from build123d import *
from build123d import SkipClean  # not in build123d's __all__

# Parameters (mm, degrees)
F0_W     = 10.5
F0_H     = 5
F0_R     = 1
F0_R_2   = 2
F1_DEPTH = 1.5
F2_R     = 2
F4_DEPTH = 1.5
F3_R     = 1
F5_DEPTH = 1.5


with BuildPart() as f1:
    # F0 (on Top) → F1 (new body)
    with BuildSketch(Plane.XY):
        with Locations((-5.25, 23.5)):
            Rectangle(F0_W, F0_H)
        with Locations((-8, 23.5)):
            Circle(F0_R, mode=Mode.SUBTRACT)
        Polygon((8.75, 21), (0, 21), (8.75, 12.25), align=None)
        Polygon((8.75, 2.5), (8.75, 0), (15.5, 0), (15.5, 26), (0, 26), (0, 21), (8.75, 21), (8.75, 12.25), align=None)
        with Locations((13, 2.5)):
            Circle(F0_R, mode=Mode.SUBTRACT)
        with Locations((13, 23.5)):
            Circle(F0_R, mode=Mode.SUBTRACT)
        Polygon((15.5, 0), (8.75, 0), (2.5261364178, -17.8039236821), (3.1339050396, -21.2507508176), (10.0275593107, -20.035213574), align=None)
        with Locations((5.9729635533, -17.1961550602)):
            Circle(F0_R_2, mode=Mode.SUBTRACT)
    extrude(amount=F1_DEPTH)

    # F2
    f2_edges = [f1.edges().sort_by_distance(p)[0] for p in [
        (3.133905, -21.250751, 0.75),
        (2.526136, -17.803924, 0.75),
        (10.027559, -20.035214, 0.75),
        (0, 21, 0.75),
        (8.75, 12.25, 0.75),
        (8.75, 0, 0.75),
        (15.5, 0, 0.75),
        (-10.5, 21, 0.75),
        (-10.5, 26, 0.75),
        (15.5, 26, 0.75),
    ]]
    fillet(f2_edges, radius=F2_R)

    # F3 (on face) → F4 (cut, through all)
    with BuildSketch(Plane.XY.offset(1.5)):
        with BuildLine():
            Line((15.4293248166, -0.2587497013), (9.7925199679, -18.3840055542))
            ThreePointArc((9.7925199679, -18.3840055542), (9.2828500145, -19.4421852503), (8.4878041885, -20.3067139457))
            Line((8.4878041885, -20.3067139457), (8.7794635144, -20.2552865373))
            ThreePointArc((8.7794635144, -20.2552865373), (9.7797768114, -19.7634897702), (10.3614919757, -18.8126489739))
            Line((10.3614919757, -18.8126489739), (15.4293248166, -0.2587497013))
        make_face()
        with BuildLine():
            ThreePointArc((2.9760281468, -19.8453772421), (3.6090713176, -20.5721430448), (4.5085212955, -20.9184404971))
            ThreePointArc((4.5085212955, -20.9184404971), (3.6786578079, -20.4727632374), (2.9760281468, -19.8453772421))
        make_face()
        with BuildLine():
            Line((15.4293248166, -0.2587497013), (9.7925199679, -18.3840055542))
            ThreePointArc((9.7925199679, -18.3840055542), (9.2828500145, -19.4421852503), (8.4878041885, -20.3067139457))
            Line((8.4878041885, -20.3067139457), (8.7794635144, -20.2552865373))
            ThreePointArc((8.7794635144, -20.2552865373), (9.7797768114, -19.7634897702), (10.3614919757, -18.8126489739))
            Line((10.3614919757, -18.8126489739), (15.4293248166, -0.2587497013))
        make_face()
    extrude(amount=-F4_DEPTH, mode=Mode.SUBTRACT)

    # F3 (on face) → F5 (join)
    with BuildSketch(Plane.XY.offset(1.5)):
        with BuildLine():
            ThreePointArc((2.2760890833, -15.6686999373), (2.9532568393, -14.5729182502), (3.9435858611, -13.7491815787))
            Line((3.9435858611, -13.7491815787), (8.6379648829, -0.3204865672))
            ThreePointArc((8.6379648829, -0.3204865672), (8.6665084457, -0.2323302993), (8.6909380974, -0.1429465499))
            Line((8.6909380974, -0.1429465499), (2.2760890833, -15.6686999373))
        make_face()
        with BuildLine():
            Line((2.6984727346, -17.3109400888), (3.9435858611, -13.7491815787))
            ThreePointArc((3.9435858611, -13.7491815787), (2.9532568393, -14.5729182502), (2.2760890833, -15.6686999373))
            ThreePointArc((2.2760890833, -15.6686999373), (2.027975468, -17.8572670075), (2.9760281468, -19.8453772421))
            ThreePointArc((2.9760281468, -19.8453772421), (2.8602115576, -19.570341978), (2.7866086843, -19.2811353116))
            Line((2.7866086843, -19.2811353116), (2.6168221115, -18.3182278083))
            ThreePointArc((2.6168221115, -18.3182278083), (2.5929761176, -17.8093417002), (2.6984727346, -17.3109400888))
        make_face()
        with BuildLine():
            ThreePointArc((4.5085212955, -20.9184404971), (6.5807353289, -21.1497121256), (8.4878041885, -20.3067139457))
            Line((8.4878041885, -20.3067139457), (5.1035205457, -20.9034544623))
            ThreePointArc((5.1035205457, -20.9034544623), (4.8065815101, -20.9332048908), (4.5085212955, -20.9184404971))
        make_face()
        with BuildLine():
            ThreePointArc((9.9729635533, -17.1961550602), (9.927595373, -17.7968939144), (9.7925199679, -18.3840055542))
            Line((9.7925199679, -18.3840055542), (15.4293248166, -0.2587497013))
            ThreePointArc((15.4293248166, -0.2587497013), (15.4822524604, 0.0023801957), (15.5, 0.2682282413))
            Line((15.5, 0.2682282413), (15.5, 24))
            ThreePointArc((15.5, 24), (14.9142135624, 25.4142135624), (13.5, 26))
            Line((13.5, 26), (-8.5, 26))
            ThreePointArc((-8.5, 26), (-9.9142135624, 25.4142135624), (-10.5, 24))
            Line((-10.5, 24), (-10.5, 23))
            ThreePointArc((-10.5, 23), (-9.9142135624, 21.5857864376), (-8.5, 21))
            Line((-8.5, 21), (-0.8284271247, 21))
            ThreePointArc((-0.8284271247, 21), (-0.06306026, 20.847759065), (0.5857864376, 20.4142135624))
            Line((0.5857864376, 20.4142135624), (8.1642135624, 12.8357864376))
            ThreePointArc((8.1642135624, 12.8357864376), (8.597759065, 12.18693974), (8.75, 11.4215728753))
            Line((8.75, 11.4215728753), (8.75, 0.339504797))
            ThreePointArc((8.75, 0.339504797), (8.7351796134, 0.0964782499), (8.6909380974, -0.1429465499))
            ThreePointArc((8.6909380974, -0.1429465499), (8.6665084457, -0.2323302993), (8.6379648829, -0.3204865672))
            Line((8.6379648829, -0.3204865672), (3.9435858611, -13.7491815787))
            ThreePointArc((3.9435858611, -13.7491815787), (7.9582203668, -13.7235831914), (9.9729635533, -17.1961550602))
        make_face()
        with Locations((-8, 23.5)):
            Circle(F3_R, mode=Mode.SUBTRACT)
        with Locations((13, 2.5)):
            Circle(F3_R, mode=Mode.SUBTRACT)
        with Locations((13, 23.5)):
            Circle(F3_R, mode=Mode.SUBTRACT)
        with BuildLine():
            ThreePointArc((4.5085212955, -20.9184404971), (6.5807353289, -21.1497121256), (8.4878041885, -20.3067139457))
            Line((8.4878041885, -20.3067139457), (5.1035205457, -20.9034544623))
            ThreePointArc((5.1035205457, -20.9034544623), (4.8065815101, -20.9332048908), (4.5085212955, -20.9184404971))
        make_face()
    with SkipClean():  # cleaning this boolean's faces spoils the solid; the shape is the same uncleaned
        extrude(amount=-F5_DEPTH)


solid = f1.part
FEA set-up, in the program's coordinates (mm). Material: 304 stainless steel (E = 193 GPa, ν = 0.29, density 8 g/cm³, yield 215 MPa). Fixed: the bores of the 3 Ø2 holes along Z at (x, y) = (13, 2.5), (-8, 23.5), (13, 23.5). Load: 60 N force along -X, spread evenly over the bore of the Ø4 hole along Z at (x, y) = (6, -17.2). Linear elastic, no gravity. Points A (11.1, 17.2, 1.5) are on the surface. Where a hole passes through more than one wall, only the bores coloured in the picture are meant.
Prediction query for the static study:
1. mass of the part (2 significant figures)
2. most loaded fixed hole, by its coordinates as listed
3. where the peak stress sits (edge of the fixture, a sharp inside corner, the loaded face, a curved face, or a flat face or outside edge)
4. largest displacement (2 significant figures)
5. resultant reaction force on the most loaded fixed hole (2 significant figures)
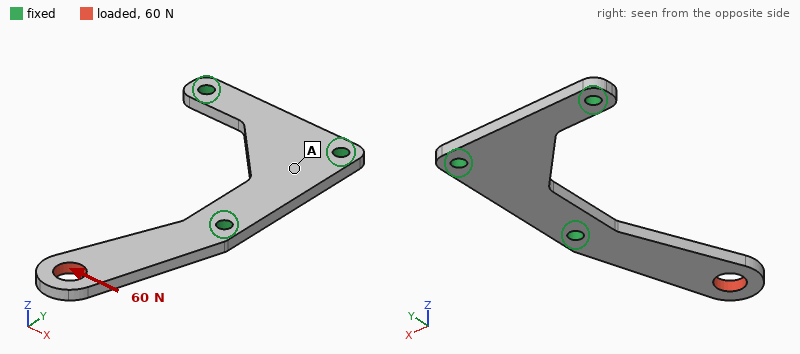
5.3 g
(13, 2.5)
edge of the fixture
41 µm
100 N
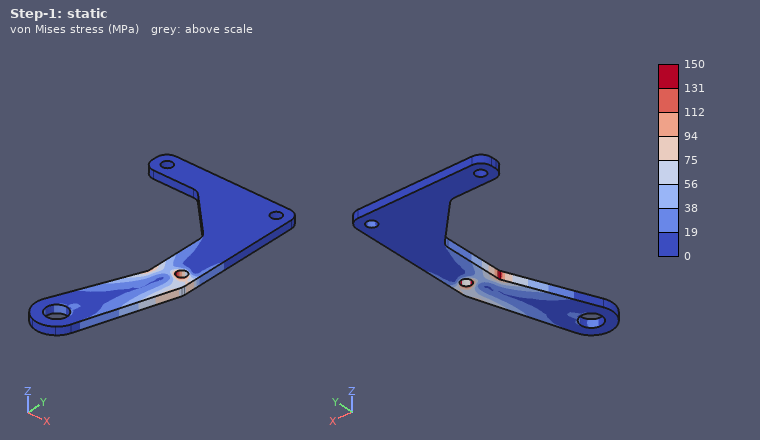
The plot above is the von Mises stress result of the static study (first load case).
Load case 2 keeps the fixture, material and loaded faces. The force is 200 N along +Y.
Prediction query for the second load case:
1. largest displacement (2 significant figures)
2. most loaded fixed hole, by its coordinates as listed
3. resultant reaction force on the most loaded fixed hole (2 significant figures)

48 µm
(13, 2.5)
150 N
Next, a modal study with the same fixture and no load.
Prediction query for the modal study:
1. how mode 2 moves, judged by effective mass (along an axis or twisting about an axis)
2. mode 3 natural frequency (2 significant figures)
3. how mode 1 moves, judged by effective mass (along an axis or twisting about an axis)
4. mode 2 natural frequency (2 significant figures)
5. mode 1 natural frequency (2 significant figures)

along X
12 kHz
along Z
7700 Hz
2200 Hz
